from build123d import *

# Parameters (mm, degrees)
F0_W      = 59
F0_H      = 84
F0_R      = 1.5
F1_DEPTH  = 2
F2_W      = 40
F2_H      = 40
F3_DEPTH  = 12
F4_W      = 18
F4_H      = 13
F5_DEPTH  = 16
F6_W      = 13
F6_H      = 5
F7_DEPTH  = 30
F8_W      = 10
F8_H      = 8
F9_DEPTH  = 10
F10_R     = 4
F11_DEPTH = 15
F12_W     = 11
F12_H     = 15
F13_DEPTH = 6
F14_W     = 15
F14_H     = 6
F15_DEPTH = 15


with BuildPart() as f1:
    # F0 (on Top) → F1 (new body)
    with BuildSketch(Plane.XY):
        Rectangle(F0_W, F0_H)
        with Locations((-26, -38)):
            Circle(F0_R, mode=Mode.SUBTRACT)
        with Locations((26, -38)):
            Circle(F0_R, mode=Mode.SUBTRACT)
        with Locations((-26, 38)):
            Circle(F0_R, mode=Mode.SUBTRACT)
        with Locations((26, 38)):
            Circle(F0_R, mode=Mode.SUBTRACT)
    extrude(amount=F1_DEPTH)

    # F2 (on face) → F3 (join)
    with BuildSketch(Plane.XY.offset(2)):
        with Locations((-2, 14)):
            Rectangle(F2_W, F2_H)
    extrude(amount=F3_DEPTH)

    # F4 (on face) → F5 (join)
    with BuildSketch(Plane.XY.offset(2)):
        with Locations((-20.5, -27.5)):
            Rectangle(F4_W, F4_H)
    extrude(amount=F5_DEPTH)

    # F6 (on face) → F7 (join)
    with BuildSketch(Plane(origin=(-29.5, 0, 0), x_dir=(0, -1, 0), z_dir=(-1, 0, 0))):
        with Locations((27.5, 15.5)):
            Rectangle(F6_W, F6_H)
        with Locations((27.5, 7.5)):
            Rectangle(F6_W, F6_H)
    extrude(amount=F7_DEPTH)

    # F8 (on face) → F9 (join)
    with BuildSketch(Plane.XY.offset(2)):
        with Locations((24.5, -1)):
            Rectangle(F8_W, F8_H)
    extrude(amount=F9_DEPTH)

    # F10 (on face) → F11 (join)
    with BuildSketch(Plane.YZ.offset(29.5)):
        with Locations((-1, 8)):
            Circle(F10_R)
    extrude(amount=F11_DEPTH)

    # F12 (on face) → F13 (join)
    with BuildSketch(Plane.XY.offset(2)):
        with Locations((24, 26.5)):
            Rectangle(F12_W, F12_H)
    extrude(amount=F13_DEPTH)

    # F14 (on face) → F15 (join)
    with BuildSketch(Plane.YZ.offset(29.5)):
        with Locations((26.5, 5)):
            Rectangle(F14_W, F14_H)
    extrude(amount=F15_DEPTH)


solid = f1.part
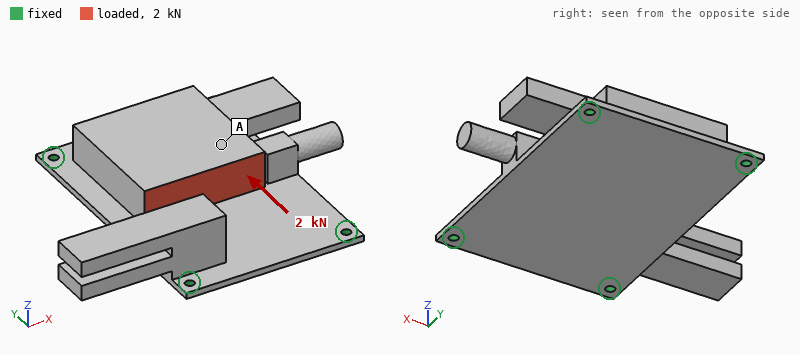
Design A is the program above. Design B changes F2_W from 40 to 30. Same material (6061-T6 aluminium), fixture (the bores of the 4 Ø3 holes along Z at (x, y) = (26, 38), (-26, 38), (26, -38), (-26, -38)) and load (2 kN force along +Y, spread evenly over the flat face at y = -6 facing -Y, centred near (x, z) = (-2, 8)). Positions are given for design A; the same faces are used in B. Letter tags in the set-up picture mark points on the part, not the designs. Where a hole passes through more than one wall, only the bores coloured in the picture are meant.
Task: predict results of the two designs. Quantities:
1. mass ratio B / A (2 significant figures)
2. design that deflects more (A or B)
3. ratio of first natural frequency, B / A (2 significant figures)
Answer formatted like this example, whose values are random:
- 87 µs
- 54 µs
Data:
- 0.88
- B
- 1.0
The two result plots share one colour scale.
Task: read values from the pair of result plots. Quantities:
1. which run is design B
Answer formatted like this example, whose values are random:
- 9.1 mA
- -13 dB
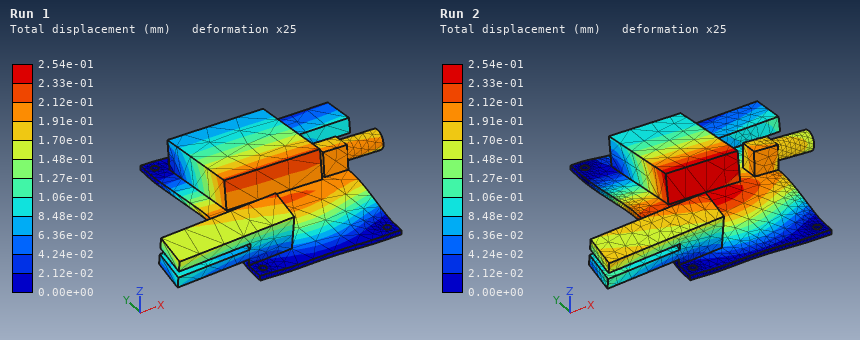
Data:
- Run 2
